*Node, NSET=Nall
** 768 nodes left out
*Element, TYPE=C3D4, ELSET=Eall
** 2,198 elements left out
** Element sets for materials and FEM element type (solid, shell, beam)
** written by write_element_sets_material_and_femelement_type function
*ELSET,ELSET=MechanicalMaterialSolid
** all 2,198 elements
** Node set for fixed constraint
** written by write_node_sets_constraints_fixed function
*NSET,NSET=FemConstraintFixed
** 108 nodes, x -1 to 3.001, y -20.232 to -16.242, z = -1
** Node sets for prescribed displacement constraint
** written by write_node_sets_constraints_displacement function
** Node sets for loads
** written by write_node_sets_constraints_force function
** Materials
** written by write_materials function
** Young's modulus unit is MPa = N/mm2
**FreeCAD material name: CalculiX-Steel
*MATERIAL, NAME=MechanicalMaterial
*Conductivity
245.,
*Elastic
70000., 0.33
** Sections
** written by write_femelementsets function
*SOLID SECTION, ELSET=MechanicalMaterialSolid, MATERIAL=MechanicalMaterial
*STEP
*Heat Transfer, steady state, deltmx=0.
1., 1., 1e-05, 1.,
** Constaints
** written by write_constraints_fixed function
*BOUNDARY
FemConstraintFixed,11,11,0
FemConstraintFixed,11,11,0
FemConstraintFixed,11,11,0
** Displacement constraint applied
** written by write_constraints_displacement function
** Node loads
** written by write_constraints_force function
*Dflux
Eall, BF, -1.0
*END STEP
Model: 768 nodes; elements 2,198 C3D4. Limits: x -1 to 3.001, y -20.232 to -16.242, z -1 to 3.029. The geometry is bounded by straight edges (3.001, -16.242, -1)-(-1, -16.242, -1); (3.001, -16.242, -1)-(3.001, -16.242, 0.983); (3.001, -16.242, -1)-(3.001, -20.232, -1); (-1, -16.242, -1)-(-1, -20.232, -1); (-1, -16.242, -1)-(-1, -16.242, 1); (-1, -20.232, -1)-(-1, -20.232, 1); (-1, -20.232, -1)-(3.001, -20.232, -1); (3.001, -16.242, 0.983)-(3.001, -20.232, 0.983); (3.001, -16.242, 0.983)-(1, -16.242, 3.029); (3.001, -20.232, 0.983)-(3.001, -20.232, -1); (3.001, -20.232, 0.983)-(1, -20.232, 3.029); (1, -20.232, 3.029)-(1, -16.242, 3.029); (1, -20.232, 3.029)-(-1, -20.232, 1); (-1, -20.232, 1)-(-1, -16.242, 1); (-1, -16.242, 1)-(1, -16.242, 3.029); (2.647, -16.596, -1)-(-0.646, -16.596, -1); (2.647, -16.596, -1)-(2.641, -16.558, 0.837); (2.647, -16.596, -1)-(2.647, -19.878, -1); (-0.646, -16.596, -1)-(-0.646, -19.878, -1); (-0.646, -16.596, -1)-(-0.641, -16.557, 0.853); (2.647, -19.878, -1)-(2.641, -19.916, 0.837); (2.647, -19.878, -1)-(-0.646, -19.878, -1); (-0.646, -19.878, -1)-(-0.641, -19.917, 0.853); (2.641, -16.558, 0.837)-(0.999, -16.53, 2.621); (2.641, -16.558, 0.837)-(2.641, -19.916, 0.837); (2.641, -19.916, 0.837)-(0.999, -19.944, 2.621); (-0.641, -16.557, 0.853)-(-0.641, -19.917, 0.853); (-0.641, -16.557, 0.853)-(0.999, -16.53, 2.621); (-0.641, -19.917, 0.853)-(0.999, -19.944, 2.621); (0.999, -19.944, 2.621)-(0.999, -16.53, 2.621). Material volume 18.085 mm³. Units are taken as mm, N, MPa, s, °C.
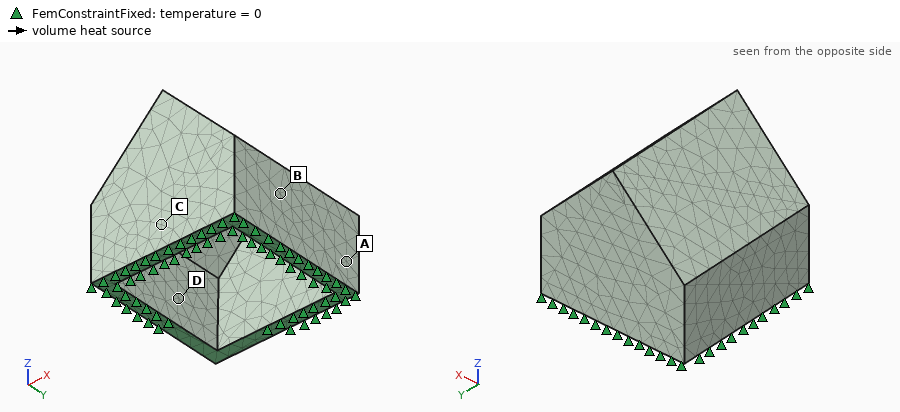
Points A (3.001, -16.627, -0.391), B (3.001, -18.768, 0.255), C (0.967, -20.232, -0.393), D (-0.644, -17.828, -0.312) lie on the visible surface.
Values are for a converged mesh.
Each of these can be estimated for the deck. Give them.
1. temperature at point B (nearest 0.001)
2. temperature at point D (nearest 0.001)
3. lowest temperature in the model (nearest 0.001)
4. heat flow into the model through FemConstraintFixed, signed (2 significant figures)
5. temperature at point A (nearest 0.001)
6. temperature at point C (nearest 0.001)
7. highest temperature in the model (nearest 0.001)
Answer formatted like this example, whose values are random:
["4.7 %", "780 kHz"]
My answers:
["-0.015 °C", "-0.009 °C", "-0.031 °C", "18 mW", "-0.008 °C", "-0.008 °C", "0.000 °C"]
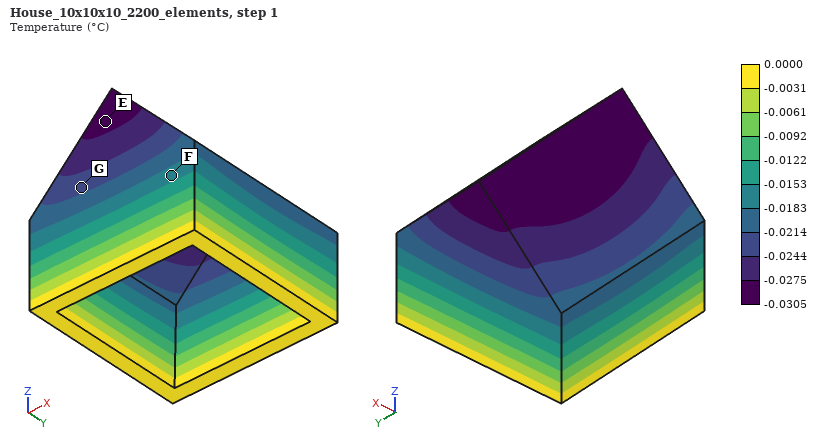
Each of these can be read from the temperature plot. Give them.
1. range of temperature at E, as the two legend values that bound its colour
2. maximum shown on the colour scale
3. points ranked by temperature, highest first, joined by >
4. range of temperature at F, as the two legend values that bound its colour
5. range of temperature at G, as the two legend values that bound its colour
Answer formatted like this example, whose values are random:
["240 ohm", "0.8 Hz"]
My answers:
["-0.0305 to -0.0275 °C", "0.0000 °C", "F > G > E", "-0.0183 to -0.0153 °C", "-0.0244 to -0.0214 °C"]
